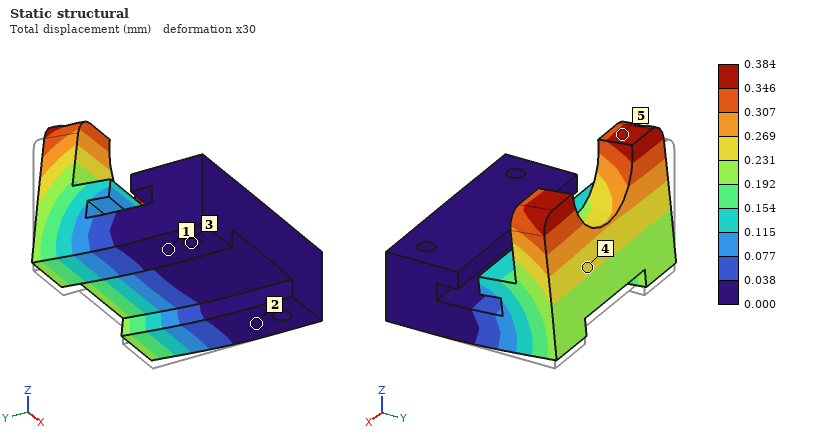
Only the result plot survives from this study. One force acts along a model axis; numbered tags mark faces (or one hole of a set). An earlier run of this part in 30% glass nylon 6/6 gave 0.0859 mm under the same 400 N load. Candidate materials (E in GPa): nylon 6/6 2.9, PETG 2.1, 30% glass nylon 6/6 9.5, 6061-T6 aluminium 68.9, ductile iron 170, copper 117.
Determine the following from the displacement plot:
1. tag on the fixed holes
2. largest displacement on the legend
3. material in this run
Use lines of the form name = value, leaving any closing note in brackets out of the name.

tag on the fixed holes = 3
largest displacement on the legend = 0.384 mm
material in this run = PETG
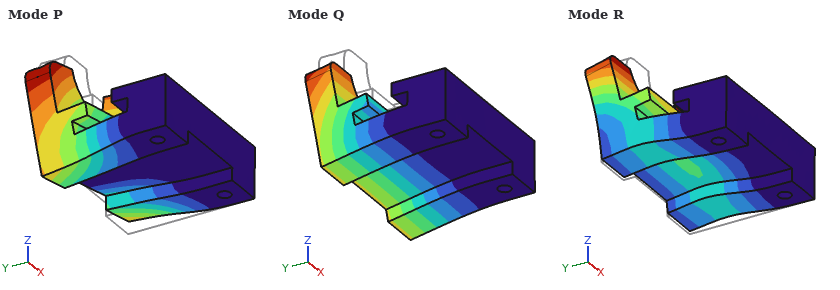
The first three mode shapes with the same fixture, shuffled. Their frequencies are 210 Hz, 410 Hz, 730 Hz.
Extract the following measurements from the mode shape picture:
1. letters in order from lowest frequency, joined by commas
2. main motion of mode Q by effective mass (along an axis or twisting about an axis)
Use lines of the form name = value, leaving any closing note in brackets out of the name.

letters in order from lowest frequency, joined by commas = Q, P, R
main motion of mode Q by effective mass = along Z
